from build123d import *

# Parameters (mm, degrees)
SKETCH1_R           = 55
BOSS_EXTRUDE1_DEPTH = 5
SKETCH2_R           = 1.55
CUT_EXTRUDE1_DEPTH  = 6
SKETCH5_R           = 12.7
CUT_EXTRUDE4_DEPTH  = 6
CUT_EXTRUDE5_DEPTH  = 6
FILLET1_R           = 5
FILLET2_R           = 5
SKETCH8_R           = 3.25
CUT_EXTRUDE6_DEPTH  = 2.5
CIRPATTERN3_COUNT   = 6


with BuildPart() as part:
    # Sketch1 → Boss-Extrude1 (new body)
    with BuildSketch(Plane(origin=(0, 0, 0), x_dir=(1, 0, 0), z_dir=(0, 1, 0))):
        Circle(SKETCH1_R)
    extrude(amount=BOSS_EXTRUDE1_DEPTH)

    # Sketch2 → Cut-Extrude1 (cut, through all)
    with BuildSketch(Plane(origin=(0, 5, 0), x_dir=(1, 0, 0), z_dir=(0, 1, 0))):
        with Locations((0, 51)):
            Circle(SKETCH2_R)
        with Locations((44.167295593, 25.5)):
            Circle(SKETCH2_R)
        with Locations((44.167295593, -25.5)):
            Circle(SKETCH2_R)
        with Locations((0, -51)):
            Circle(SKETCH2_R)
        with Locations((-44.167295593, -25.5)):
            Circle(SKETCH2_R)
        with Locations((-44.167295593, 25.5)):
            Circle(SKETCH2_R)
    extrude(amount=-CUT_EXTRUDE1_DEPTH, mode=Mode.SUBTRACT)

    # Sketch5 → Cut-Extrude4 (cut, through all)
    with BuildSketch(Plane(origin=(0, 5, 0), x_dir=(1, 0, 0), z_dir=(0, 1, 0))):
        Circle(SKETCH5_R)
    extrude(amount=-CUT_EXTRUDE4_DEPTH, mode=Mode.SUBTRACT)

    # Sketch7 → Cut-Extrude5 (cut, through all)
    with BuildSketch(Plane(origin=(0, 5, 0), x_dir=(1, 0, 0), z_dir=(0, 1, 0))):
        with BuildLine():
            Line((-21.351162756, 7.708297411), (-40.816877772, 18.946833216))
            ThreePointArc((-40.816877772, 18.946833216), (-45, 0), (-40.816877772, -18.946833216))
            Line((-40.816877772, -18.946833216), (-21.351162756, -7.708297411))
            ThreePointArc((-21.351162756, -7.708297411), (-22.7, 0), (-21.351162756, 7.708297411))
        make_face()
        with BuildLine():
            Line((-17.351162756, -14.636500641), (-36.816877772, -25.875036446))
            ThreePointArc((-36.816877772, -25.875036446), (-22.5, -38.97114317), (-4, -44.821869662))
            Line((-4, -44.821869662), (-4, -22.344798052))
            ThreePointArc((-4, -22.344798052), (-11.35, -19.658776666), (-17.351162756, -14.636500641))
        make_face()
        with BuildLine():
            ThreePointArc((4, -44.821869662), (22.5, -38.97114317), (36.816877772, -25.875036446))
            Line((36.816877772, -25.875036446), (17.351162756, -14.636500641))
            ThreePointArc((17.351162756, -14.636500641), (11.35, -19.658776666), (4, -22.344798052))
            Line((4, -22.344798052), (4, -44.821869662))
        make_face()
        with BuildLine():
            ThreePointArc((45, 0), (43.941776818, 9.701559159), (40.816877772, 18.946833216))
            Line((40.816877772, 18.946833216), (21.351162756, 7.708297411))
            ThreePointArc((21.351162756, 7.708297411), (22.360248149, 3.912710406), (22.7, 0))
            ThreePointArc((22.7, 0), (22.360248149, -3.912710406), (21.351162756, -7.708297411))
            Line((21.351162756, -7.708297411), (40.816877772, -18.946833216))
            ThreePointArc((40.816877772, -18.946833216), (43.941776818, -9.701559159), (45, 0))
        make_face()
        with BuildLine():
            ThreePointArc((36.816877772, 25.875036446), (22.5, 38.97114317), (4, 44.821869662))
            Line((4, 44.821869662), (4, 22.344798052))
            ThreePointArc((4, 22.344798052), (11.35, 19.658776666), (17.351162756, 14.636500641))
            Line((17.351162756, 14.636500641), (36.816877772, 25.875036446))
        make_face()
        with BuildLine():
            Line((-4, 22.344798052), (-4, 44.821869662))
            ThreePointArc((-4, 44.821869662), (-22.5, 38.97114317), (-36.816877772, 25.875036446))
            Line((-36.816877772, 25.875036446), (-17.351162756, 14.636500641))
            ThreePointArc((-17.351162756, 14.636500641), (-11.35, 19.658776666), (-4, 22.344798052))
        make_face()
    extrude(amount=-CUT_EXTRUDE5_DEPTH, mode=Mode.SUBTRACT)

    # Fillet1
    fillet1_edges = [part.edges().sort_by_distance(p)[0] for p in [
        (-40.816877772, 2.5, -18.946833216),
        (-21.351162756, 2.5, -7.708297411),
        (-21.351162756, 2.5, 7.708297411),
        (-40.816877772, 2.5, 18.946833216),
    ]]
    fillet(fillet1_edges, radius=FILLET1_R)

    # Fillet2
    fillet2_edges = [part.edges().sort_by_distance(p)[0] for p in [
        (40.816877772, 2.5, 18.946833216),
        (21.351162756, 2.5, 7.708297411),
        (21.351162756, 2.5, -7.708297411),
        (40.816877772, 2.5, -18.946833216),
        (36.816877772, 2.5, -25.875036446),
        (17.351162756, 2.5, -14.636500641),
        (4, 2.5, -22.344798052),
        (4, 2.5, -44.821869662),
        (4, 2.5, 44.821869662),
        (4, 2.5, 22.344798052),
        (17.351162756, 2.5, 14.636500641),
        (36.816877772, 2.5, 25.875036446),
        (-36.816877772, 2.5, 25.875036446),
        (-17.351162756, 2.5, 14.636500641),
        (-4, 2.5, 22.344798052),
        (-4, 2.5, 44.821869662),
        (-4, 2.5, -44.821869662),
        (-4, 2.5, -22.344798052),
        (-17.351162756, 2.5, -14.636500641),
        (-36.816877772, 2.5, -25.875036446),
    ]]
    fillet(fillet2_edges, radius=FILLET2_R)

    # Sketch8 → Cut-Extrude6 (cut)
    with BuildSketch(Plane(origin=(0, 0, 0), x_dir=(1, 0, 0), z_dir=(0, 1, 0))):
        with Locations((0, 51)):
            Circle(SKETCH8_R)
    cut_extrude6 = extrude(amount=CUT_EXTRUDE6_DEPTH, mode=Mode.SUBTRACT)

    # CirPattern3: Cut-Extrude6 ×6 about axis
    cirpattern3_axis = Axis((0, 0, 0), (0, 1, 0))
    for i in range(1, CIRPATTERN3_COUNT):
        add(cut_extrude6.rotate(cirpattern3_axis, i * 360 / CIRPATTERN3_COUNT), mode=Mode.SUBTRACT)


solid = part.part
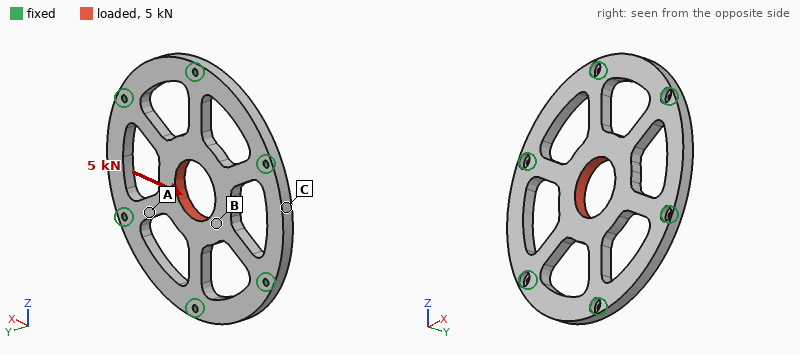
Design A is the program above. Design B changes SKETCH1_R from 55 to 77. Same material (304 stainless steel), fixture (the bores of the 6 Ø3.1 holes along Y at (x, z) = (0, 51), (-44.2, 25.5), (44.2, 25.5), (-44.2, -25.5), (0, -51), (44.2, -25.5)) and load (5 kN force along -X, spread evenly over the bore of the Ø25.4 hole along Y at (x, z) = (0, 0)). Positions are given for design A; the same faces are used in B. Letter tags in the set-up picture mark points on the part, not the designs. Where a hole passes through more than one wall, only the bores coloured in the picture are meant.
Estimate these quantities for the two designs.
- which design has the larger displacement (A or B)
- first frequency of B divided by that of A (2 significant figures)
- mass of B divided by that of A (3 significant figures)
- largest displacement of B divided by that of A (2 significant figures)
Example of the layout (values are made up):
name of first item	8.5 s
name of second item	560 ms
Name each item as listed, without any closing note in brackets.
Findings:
which design has the larger displacement	A
first frequency of B divided by that of A	0.82
mass of B divided by that of A	2.71
largest displacement of B divided by that of A	0.90
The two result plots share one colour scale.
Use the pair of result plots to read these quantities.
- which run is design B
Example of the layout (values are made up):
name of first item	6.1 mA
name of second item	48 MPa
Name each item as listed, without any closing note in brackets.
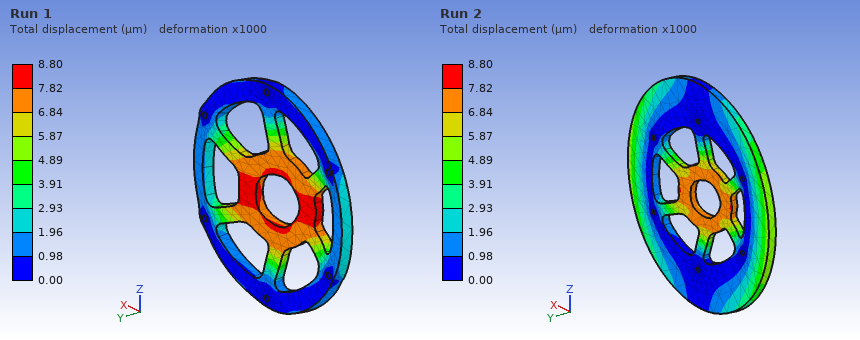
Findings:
which run is design B	Run 2
